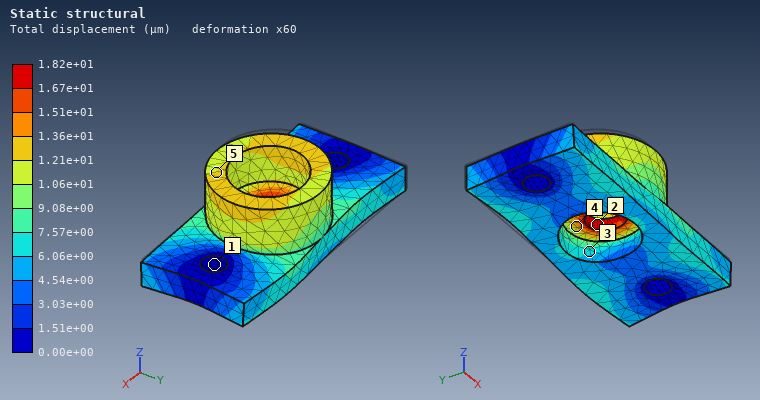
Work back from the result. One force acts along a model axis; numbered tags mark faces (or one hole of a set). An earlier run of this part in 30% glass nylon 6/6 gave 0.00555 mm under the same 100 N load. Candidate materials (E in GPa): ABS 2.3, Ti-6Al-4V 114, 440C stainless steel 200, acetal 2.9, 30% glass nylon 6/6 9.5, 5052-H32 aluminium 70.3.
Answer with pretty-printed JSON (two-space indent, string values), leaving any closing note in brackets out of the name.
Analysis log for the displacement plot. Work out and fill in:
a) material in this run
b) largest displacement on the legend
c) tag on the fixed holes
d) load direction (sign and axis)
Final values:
{
  "material in this run": "acetal",
  "largest displacement on the legend": "1.82e+01 µm",
  "tag on the fixed holes": "1",
  "load direction": "+X"
}
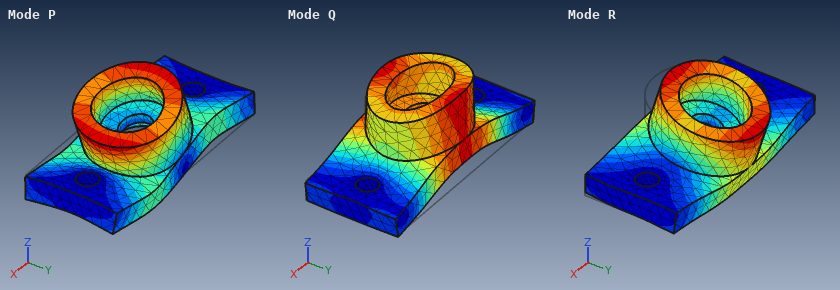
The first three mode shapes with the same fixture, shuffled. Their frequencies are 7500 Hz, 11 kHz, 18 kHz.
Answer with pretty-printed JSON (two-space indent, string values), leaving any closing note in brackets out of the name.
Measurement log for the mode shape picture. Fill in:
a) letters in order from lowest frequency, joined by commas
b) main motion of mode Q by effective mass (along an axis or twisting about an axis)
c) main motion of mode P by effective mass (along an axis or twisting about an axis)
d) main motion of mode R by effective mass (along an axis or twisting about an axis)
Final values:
{
  "letters in order from lowest frequency, joined by commas": "R, Q, P",
  "main motion of mode Q by effective mass": "along Z",
  "main motion of mode P by effective mass": "along X",
  "main motion of mode R by effective mass": "along Y"
}
